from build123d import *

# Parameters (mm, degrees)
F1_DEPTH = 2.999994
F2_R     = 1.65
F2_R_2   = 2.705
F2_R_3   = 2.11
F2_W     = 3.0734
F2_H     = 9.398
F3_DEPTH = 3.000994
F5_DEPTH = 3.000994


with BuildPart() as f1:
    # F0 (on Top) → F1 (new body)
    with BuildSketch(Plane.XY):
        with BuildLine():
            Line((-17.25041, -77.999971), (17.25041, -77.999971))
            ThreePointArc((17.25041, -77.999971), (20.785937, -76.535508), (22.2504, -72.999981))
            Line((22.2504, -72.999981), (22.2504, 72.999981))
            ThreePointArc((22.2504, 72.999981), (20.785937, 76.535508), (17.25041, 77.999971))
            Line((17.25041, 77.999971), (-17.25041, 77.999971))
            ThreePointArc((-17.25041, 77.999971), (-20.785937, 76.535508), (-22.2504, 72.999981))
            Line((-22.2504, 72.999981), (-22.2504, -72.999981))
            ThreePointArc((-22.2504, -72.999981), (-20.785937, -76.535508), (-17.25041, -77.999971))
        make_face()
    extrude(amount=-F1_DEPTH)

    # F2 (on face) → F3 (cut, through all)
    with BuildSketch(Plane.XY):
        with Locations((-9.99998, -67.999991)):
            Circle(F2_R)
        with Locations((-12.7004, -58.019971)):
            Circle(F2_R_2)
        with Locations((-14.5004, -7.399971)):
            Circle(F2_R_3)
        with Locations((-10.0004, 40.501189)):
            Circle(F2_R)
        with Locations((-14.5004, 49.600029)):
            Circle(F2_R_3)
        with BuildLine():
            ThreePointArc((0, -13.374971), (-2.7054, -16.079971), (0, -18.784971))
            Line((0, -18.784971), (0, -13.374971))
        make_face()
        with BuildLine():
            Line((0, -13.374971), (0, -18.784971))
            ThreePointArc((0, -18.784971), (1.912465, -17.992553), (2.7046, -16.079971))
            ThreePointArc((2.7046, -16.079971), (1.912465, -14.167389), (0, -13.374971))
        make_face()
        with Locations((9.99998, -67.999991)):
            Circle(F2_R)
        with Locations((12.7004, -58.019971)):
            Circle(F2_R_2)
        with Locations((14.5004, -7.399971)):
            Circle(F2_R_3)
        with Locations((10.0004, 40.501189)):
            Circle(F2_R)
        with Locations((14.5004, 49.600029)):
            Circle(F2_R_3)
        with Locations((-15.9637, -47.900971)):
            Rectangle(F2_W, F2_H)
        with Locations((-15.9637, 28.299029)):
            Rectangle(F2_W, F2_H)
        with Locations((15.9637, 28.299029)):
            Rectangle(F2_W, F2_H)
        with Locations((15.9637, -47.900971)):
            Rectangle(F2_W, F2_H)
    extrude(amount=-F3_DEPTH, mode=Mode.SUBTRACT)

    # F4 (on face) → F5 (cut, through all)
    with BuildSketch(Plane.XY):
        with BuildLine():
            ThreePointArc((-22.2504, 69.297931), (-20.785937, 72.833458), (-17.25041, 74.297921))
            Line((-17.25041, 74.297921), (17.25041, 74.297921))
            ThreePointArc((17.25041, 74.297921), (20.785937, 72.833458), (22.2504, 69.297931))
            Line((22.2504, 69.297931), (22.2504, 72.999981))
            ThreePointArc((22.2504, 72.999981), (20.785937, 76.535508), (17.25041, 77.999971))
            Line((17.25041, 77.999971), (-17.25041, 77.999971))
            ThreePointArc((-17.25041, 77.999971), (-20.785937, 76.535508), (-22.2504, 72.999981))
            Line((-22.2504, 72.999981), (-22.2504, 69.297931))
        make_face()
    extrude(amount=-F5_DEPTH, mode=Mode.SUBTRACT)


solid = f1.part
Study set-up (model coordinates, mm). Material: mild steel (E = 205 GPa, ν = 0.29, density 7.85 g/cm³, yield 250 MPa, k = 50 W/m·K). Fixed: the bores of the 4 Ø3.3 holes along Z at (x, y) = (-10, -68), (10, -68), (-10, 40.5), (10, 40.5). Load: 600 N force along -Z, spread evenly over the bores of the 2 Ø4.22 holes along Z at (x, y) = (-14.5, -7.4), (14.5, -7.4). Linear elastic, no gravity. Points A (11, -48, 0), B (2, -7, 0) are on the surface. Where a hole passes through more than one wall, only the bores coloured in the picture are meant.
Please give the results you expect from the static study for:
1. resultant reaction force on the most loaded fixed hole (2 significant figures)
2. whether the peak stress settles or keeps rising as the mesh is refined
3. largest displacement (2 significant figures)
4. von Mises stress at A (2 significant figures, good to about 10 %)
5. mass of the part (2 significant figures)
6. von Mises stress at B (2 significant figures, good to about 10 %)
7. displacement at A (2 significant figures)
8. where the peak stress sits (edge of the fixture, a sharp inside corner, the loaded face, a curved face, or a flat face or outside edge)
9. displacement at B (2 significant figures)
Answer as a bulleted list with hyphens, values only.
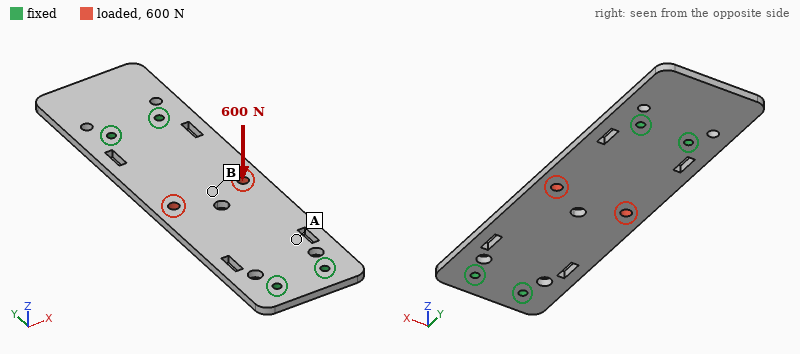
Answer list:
- 180 N
- keeps rising
- 0.22 mm
- 30 MPa
- 150 g
- 110 MPa
- 0.064 mm
- edge of the fixture
- 0.20 mm
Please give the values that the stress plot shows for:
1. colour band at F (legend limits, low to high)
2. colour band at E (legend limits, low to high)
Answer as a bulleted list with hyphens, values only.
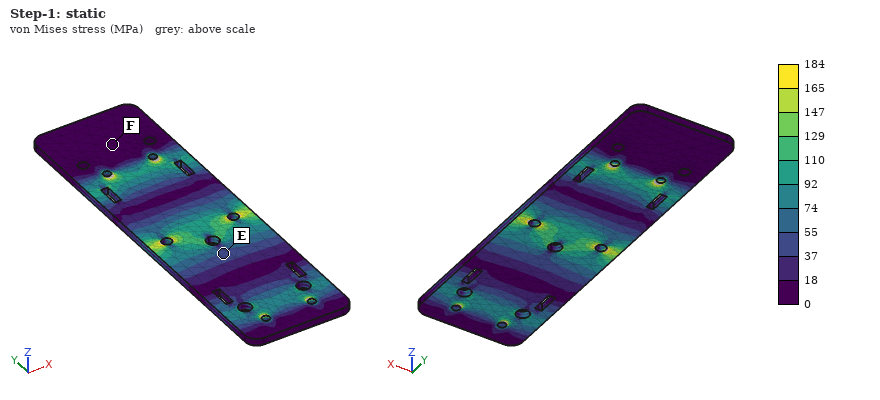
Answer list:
- 0 to 18 MPa
- 37 to 55 MPa
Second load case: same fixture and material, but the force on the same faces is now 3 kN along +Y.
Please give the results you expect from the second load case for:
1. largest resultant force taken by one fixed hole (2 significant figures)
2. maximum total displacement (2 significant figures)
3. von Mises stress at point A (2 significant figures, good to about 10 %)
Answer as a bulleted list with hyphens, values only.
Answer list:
- 850 N
- 4.3 µm
- 11 MPa
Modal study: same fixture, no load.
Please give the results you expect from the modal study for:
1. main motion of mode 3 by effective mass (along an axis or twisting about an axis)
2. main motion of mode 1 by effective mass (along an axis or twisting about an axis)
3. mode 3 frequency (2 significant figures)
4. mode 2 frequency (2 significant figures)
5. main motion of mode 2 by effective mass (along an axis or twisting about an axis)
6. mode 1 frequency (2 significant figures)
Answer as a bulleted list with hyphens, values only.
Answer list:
- twisting about Y
- along Z
- 2300 Hz
- 2100 Hz
- along Z
- 1300 Hz
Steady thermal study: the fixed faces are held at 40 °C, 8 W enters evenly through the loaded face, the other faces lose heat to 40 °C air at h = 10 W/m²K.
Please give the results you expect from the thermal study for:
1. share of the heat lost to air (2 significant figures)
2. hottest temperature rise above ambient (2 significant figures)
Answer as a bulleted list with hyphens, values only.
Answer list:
- 21 %
- 34 K
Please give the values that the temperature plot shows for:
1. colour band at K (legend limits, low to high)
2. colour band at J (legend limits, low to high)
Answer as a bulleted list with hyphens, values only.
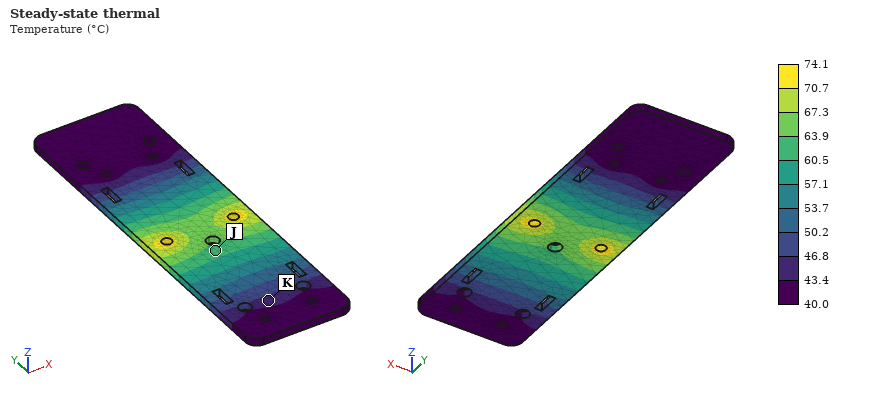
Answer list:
- 43.4 to 46.8 °C
- 60.5 to 63.9 °C
